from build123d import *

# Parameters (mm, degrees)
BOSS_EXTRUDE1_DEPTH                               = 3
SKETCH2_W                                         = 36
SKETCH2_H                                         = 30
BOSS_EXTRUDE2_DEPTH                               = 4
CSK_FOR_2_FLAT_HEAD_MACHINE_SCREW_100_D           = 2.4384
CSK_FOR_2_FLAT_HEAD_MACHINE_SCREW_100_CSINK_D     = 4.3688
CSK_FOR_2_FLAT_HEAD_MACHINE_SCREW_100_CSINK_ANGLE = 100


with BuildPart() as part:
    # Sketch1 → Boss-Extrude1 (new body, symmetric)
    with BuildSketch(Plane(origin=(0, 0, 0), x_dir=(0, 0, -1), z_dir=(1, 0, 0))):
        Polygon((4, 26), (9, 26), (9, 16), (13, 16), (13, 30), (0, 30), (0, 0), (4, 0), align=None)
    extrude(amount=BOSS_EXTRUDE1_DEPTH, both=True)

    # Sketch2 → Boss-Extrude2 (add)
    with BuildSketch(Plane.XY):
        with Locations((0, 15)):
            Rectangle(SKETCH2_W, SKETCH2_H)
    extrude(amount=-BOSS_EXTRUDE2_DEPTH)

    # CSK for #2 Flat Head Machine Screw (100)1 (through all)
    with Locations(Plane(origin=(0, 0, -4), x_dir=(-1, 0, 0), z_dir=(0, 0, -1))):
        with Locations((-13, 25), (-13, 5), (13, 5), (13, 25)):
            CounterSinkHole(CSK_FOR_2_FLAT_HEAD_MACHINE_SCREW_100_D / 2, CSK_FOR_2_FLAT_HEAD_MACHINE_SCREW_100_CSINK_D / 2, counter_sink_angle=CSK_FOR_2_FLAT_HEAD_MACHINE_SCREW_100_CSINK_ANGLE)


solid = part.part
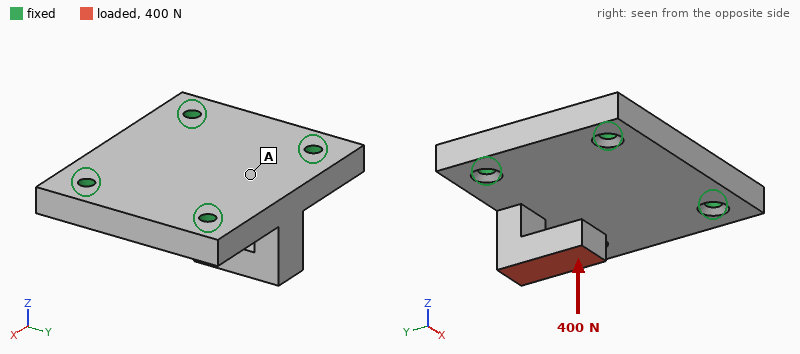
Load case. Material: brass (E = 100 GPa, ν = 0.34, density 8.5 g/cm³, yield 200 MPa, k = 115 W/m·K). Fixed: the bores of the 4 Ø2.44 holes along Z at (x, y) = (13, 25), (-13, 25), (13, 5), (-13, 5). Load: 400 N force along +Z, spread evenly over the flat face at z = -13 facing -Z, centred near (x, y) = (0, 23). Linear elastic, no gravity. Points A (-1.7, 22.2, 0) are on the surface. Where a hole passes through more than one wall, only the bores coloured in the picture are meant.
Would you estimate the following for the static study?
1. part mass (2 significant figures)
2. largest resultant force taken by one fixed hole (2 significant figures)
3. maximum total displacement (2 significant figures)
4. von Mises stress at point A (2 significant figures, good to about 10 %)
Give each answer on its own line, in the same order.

40 g
190 N
92 µm
23 MPa
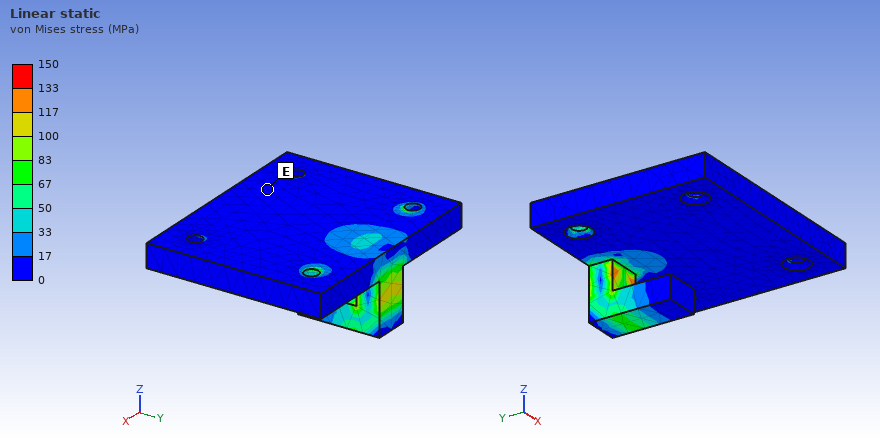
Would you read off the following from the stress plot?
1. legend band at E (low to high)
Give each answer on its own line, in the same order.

0 to 17 MPa
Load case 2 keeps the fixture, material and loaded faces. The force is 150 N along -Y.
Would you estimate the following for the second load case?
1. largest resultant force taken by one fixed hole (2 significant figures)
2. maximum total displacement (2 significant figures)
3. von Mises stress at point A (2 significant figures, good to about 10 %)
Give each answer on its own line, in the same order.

62 N
51 µm
15 MPa
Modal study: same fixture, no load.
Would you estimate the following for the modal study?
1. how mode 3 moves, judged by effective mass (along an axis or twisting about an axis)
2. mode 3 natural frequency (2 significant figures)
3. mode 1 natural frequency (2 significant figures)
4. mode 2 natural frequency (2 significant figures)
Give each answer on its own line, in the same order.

along Z
11 kHz
6100 Hz
7400 Hz
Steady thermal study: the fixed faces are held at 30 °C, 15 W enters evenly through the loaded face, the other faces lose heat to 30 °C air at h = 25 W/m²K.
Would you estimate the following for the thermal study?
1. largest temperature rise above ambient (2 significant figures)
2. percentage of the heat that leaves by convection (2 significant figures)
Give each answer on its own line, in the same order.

80 K
4.5 %
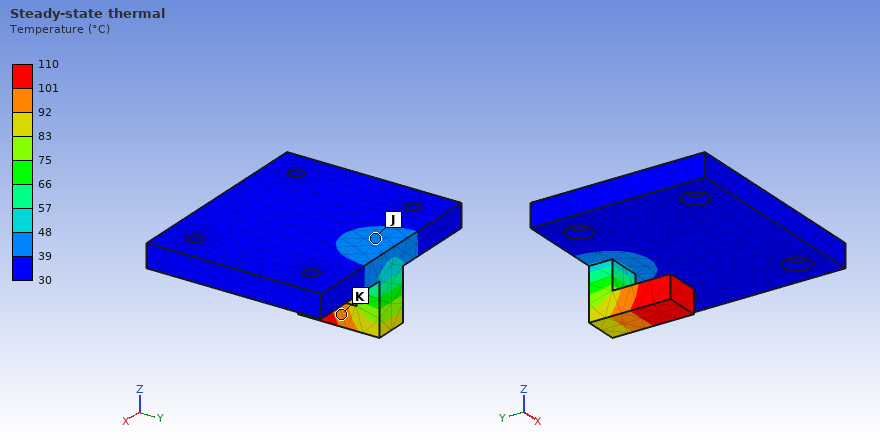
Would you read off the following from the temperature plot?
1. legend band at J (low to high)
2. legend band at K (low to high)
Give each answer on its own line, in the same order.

39 to 48 °C
92 to 101 °C
